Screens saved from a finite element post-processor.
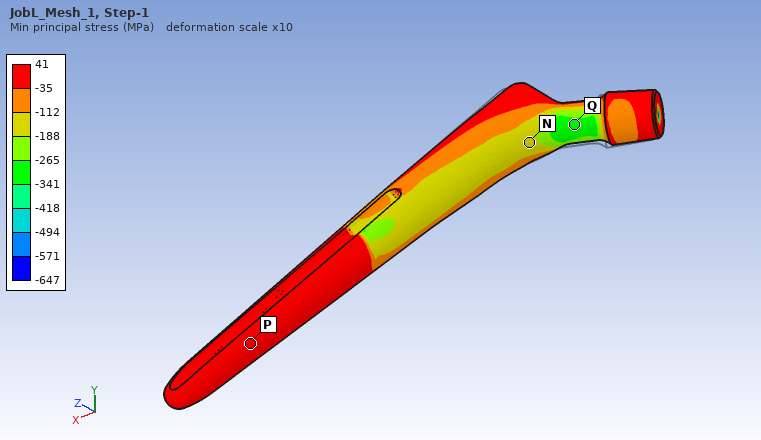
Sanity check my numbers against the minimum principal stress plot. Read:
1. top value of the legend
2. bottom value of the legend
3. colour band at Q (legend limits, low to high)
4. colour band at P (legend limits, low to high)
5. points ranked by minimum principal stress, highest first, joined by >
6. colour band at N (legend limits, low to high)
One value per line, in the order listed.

41 MPa
-647 MPa
-341 to -265 MPa
-35 to 41 MPa
P > N > Q
-188 to -112 MPa
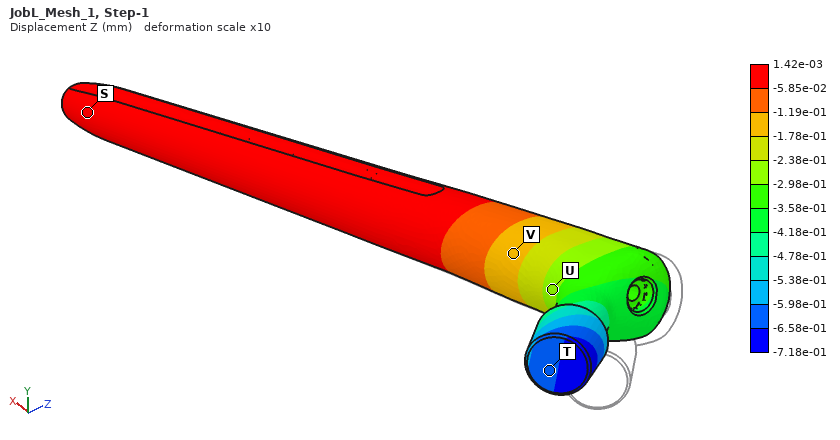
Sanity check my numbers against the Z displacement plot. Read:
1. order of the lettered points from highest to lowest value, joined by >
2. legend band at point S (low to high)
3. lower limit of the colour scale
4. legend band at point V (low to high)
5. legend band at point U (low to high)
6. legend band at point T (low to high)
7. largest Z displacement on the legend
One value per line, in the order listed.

S > V > U > T
-5.85e-02 to 1.42e-03 mm
-7.18e-01 mm
-1.78e-01 to -1.19e-01 mm
-2.98e-01 to -2.38e-01 mm
-6.58e-01 to -5.98e-01 mm
1.42e-03 mm
